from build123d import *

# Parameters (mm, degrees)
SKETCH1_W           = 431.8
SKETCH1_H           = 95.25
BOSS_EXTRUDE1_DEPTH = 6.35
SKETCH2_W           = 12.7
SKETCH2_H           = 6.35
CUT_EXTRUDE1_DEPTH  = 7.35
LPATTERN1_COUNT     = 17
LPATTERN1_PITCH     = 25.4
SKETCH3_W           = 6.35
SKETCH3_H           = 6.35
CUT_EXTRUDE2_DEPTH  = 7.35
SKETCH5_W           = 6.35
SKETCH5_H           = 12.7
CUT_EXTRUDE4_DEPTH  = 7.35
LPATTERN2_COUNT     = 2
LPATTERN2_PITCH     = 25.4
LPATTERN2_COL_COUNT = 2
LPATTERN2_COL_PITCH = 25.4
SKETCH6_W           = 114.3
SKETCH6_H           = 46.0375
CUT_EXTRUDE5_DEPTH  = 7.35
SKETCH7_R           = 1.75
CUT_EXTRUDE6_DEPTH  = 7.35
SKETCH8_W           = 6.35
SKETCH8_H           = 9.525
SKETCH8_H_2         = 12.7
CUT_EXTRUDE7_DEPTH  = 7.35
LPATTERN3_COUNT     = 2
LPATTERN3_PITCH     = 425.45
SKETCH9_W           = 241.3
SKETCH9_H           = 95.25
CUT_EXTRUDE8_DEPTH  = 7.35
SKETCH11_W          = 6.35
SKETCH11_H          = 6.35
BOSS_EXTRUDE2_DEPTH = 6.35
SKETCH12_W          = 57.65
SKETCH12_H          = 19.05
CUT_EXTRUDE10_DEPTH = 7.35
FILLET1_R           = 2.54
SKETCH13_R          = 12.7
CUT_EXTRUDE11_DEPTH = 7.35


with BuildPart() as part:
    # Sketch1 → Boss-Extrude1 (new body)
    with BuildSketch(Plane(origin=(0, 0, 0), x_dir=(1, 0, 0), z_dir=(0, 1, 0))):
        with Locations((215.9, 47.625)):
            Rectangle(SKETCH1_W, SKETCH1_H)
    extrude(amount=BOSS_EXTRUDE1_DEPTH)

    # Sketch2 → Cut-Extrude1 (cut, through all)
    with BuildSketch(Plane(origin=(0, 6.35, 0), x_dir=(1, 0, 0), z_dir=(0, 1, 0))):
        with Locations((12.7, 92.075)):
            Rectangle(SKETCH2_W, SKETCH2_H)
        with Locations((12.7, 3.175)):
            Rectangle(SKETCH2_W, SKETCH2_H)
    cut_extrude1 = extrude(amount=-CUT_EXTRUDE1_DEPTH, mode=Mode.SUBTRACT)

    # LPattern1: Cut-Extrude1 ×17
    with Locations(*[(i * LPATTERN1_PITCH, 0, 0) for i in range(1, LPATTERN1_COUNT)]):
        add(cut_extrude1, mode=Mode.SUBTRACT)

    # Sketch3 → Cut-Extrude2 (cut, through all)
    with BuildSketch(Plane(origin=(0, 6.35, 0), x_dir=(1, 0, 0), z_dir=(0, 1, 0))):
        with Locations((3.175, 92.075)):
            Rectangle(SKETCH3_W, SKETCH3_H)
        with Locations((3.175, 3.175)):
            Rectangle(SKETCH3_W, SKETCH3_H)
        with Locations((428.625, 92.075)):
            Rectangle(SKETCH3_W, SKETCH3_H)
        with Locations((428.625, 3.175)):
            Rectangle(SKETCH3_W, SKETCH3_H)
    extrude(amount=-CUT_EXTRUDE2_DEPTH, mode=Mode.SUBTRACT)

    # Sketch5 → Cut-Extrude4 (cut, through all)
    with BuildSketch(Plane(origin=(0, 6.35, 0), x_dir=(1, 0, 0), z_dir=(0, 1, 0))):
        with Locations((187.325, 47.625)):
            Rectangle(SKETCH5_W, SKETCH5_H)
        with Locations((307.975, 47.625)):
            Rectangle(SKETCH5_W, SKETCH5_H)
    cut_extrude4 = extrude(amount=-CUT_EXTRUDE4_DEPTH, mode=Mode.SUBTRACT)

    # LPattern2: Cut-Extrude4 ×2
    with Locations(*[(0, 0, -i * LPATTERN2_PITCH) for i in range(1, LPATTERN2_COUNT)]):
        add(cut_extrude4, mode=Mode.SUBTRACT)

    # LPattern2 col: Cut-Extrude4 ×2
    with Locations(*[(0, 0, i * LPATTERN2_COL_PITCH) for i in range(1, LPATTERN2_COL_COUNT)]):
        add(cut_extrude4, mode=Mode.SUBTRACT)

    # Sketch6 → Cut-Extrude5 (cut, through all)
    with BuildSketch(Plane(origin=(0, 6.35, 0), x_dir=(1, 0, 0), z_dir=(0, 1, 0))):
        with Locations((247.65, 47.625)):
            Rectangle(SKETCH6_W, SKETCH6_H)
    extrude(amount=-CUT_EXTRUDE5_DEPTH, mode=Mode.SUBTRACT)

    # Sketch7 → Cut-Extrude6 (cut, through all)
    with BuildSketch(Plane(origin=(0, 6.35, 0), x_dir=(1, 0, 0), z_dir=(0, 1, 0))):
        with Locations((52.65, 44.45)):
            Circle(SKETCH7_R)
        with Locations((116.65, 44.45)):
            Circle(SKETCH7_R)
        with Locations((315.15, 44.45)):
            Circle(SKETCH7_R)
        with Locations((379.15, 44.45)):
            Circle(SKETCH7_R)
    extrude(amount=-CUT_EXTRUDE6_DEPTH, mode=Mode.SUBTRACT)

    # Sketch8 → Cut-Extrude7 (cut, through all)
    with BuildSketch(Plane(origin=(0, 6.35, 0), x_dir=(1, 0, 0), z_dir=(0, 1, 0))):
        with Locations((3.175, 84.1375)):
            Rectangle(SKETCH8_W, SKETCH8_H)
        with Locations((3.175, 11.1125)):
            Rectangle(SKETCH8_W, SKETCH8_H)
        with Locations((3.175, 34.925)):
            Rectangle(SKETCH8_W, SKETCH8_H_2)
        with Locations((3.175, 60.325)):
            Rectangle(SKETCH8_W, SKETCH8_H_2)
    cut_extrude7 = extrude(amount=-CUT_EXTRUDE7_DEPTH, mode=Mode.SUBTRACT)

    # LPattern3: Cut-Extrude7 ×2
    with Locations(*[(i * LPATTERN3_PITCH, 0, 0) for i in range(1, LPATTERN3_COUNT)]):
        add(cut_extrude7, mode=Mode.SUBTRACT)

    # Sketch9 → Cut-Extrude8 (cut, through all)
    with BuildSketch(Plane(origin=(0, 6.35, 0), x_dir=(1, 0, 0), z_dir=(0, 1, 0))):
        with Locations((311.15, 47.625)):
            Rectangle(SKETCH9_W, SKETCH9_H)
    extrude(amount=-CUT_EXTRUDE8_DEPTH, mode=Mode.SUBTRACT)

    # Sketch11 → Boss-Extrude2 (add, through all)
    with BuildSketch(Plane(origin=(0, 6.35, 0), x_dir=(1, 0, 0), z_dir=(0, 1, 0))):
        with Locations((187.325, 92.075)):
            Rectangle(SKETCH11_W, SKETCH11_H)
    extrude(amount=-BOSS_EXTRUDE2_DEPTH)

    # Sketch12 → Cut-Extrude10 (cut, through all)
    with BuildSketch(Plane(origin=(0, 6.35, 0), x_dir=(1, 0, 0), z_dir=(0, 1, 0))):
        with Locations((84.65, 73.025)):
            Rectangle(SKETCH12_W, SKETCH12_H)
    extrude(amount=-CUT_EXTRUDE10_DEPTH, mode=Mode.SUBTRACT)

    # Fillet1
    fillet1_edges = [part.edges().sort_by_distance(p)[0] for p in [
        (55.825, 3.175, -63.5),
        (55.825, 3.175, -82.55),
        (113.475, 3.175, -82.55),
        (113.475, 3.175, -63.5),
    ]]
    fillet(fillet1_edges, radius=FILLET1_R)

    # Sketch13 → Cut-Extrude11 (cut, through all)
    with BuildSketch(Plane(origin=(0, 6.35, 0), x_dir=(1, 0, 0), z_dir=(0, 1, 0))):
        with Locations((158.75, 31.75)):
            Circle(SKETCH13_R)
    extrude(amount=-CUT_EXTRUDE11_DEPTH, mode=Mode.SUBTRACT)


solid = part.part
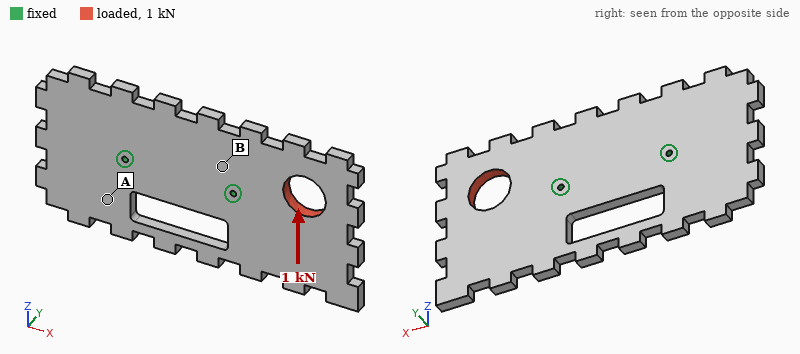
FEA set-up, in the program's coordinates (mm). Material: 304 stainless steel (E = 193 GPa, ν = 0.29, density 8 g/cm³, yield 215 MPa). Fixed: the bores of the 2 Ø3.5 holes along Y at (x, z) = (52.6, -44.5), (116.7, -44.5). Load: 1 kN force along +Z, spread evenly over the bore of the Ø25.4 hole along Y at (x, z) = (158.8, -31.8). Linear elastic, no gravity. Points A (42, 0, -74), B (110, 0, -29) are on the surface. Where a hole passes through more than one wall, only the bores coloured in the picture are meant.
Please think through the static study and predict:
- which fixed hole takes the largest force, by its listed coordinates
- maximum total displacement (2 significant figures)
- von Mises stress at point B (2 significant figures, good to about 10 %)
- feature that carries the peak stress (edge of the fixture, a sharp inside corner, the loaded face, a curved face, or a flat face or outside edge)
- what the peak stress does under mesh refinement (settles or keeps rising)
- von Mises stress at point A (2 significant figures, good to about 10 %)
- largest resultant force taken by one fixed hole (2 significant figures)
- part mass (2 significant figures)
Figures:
(116.7, -44.5)
11 µm
4.8 MPa
edge of the fixture
keeps rising
1.9 MPa
1.6 kN
750 g
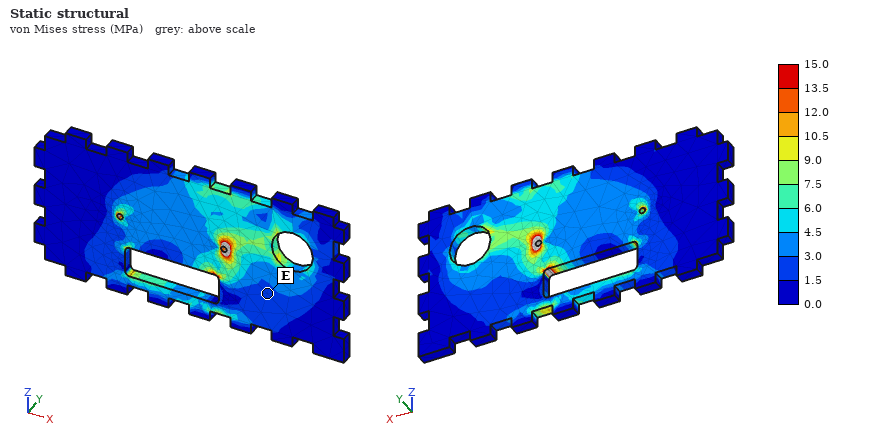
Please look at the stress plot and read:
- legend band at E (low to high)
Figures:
1.5 to 3.0 MPa
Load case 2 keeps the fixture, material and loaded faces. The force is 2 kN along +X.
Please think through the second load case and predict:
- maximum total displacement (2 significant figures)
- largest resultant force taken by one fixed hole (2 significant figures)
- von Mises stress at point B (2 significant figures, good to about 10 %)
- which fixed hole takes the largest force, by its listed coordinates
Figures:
5.4 µm
1.5 kN
5.2 MPa
(116.7, -44.5)
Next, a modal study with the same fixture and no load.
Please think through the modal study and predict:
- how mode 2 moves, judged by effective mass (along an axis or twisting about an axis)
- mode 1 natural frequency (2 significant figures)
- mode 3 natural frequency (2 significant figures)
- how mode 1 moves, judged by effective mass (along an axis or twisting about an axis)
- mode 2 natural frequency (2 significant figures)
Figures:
twisting about X
740 Hz
1300 Hz
along Y
1000 Hz
